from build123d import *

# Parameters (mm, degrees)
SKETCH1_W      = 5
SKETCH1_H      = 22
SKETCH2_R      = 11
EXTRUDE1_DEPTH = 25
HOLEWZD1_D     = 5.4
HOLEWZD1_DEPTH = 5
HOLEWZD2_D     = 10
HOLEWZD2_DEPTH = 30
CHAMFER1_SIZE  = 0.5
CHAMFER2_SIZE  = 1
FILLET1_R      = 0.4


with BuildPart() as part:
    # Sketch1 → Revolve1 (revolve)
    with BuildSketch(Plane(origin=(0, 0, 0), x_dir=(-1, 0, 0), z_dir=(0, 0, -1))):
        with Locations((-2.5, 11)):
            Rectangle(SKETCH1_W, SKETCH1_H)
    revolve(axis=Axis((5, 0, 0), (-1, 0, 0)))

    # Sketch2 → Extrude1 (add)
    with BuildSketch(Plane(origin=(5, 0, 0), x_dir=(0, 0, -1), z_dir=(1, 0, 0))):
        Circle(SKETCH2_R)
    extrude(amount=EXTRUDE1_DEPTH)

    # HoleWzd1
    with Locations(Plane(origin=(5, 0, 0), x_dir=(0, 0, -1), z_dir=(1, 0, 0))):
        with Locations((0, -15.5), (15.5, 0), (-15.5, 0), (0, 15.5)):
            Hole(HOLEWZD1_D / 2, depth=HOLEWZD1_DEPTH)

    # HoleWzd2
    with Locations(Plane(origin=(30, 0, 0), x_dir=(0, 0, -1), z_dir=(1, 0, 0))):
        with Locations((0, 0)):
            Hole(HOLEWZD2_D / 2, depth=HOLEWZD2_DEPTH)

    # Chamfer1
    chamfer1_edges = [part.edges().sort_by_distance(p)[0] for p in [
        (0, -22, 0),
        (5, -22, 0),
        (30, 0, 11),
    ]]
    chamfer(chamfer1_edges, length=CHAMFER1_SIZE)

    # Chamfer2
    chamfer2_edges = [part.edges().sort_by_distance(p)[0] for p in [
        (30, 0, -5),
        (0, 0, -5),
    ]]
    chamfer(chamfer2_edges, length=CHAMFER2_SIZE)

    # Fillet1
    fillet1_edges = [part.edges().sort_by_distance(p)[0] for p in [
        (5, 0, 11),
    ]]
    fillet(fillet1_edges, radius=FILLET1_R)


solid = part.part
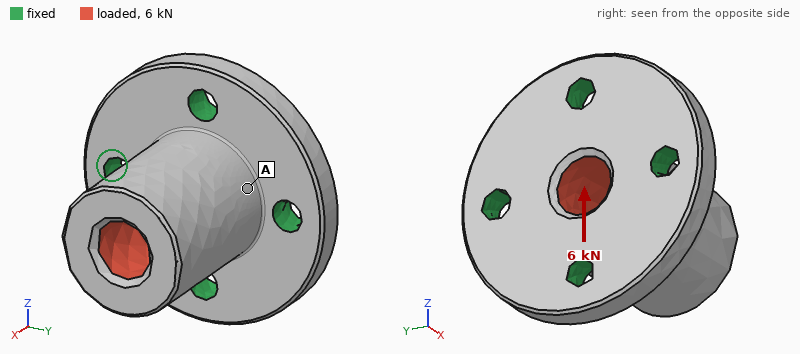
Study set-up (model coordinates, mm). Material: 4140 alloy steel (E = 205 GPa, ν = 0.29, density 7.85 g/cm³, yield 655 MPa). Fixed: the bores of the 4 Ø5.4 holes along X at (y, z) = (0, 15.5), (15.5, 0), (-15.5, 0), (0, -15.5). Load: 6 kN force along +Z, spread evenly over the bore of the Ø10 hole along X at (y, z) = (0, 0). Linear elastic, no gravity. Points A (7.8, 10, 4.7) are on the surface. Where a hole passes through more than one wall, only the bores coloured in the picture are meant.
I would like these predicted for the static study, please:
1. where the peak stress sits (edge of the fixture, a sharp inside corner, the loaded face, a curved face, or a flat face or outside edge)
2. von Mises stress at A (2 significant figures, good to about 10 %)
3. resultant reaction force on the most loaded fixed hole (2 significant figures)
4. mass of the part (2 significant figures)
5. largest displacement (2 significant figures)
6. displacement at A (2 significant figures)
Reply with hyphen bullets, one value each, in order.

- a curved face
- 27 MPa
- 3.4 kN
- 110 g
- 18 µm
- 3.5 µm
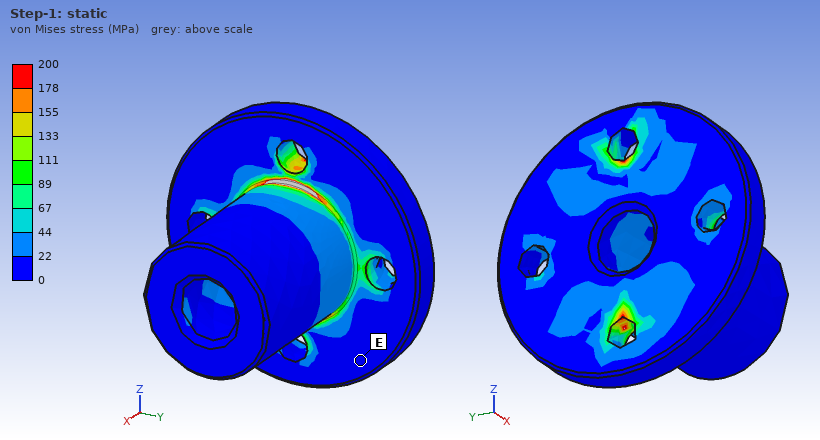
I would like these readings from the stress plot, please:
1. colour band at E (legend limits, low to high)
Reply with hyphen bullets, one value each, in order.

- 0 to 22 MPa
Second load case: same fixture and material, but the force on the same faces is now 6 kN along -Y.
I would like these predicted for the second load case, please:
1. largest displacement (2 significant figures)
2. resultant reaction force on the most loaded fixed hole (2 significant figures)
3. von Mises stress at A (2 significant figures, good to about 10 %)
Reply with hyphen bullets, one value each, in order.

- 18 µm
- 3.4 kN
- 53 MPa
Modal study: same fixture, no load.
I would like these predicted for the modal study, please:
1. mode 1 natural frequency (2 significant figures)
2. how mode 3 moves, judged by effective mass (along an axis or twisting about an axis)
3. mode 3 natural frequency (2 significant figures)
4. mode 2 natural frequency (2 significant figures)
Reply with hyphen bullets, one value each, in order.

- 13 kHz
- along X
- 26 kHz
- 13 kHz
